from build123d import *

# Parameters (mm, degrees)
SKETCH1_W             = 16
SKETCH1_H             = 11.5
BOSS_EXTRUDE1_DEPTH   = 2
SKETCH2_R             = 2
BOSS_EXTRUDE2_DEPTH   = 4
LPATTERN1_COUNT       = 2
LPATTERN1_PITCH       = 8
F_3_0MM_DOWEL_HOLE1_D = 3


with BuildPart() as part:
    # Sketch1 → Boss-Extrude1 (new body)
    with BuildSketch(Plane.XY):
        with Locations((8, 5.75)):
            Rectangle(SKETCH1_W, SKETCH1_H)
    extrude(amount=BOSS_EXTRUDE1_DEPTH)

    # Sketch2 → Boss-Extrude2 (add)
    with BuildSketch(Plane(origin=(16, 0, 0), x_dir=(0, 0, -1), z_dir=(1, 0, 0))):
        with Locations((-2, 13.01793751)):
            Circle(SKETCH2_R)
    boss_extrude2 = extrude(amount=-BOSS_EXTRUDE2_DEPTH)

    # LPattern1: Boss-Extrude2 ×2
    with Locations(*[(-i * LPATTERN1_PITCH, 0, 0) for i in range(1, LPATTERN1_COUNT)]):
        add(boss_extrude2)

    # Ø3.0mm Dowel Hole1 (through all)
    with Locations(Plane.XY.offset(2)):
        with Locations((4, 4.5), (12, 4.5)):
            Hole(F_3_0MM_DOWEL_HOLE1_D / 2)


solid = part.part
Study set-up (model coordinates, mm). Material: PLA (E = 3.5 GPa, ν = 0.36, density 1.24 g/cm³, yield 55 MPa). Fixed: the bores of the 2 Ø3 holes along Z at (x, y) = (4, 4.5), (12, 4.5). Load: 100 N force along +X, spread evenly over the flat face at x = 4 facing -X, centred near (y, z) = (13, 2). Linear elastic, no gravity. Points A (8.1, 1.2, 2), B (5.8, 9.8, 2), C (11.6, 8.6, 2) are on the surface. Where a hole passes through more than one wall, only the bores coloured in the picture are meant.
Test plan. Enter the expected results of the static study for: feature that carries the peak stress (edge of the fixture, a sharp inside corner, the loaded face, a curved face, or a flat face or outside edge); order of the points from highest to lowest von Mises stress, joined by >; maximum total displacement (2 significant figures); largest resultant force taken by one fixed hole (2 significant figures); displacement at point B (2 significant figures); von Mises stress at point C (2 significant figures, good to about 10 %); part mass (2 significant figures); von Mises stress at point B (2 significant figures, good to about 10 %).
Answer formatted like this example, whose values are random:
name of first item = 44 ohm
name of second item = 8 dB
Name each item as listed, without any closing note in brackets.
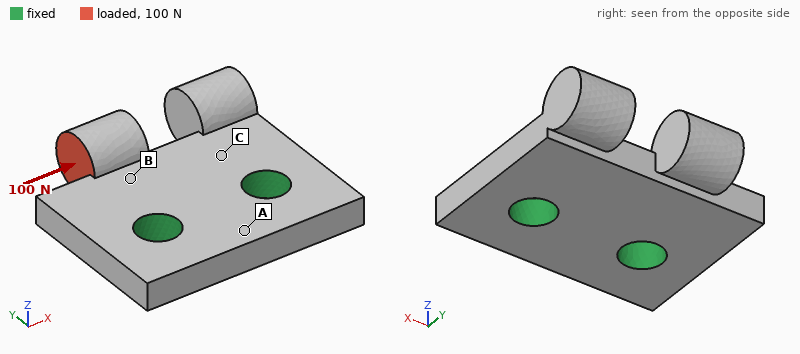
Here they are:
feature that carries the peak stress = a flat face or outside edge
order of the points from highest to lowest von Mises stress, joined by > = B > C > A
maximum total displacement = 0.12 mm
largest resultant force taken by one fixed hole = 99 N
displacement at point B = 0.025 mm
von Mises stress at point C = 7.1 MPa
part mass = 0.54 g
von Mises stress at point B = 11 MPa
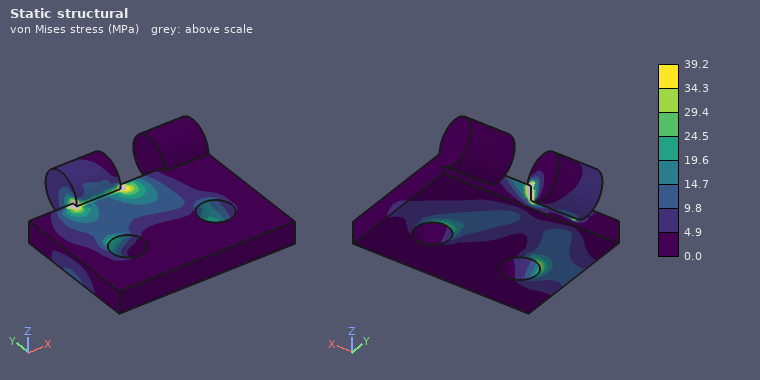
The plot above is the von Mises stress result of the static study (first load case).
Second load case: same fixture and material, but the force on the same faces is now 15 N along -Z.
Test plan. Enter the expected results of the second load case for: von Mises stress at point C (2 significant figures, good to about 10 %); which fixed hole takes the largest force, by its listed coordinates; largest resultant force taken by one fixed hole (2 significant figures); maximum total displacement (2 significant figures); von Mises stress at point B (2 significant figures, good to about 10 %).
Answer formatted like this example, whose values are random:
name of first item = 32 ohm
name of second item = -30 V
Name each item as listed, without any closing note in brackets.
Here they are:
von Mises stress at point C = 4.9 MPa
which fixed hole takes the largest force, by its listed coordinates = (4, 4.5)
largest resultant force taken by one fixed hole = 14 N
maximum total displacement = 0.17 mm
von Mises stress at point B = 12 MPa
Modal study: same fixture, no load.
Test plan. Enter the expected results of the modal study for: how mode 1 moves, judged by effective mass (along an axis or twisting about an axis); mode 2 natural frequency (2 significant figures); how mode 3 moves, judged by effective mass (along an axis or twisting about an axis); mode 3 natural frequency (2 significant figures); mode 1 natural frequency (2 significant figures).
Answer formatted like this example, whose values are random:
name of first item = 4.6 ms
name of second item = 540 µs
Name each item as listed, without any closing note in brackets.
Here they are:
how mode 1 moves, judged by effective mass = along Z
mode 2 natural frequency = 7300 Hz
how mode 3 moves, judged by effective mass = along X
mode 3 natural frequency = 15 kHz
mode 1 natural frequency = 5600 Hz
